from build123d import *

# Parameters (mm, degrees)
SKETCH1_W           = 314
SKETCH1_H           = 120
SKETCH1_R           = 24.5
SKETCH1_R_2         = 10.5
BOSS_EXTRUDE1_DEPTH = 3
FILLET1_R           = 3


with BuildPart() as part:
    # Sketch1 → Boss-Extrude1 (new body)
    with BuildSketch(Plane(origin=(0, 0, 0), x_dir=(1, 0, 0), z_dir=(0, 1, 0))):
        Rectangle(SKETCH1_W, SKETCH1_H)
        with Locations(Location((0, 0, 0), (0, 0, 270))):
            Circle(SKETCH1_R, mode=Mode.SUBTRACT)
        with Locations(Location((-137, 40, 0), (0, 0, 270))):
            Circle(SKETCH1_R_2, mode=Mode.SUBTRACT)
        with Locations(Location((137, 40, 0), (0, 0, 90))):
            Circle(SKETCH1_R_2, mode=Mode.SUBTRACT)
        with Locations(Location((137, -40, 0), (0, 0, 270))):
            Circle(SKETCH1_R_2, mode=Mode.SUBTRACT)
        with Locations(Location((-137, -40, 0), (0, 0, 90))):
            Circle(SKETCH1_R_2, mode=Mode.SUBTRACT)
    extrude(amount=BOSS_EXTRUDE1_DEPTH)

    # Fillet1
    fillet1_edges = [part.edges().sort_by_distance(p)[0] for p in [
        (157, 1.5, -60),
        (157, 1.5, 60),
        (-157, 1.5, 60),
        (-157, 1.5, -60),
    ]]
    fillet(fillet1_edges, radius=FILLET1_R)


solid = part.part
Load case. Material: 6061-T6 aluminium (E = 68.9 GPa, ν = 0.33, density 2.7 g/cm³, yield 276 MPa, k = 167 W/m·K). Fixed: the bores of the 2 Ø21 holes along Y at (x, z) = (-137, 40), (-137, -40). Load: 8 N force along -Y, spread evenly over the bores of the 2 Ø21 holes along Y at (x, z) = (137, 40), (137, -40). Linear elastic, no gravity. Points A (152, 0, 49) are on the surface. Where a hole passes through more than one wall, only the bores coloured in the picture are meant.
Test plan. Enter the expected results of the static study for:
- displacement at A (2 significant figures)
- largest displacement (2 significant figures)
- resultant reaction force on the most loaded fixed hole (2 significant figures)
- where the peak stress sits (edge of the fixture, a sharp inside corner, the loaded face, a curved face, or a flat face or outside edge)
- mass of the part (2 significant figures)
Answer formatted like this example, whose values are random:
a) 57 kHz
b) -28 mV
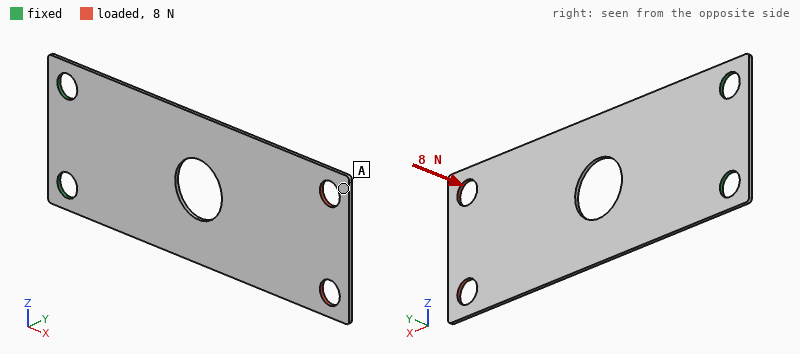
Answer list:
a) 3.2 mm
b) 3.3 mm
c) 4.0 N
d) a flat face or outside edge
e) 280 g
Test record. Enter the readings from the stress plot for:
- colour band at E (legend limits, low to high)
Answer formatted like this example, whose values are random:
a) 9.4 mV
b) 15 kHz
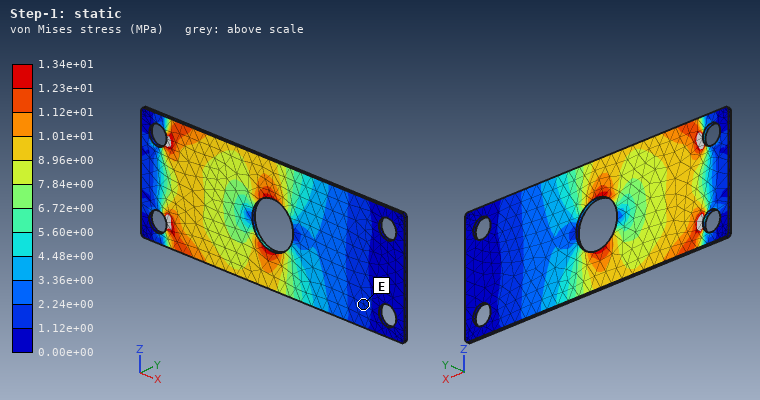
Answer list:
a) 1.12e+00 to 2.24e+00 MPa
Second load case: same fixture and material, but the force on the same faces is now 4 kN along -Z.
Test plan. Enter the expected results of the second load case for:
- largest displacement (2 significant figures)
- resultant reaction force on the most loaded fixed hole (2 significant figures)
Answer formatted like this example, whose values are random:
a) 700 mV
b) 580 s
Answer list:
a) 1.2 mm
b) 12 kN
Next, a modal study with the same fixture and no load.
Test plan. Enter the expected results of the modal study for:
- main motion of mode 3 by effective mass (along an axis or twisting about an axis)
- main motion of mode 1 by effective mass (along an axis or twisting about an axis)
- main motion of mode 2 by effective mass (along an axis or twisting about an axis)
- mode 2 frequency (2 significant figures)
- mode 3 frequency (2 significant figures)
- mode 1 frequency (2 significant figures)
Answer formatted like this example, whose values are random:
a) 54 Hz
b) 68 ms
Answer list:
a) along Y
b) along Y
c) twisting about X
d) 150 Hz
e) 190 Hz
f) 30 Hz
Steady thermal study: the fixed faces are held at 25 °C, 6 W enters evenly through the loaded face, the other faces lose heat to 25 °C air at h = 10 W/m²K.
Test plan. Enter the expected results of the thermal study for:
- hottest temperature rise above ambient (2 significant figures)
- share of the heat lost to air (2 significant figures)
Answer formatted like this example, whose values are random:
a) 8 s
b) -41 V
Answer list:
a) 16 K
b) 71 %
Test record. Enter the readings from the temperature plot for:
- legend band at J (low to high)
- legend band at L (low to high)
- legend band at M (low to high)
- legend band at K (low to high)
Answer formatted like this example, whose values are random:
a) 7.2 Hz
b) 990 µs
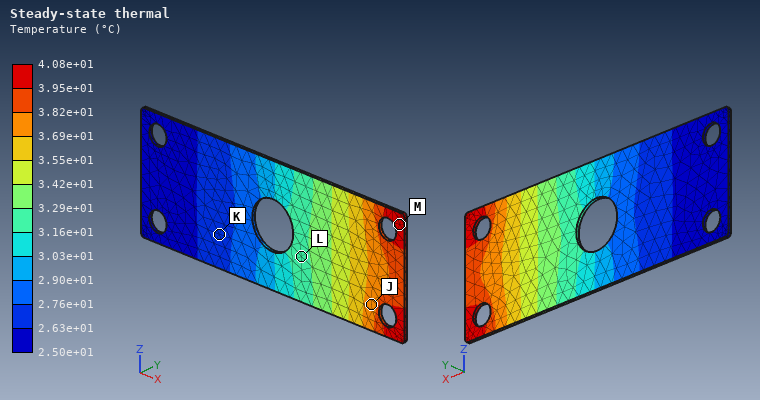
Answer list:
a) 3.69e+01 to 3.82e+01 °C
b) 3.16e+01 to 3.29e+01 °C
c) 3.95e+01 to 4.08e+01 °C
d) 2.63e+01 to 2.76e+01 °C
